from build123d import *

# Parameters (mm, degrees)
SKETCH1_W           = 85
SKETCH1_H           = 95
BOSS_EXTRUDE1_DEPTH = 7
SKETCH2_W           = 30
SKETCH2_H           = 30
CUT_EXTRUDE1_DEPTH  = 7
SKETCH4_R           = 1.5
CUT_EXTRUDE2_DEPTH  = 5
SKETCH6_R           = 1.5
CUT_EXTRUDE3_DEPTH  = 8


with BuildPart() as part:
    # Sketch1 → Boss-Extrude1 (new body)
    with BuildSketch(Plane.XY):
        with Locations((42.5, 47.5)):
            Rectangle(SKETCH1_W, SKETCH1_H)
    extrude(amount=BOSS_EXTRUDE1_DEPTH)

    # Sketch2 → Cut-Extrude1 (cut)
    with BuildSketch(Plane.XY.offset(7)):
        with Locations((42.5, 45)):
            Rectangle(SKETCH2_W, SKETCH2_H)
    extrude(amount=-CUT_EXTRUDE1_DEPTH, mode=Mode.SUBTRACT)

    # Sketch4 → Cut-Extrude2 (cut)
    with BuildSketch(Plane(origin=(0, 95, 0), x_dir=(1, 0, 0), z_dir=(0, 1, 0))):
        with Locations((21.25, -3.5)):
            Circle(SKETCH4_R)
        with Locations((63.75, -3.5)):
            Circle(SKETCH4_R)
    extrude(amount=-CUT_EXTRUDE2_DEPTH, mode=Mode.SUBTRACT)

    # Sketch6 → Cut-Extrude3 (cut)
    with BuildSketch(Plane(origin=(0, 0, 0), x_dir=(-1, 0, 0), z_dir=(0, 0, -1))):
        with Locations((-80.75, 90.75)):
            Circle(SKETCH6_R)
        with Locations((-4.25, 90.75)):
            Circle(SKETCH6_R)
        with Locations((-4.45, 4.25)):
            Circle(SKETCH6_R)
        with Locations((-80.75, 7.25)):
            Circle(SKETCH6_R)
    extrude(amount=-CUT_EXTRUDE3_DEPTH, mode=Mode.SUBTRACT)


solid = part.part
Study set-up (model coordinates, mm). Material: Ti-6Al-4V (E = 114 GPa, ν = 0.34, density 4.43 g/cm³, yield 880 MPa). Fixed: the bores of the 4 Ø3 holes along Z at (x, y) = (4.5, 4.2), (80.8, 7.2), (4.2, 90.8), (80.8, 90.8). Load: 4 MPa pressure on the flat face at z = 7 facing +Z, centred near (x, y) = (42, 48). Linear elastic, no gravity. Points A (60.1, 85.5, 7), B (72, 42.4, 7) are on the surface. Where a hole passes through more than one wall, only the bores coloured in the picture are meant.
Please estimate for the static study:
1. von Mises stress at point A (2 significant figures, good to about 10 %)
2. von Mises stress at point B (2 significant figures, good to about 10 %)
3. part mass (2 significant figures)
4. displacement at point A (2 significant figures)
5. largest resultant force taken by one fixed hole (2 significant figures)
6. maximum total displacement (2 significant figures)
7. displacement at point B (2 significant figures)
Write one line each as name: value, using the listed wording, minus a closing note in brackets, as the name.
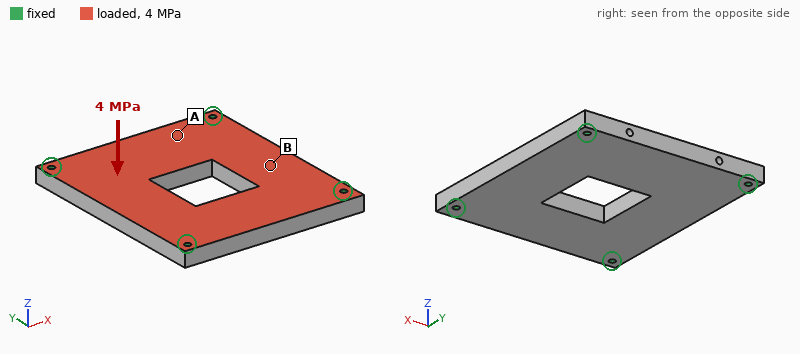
von Mises stress at point A: 110 MPa
von Mises stress at point B: 200 MPa
part mass: 220 g
displacement at point A: 0.20 mm
largest resultant force taken by one fixed hole: 7.5 kN
maximum total displacement: 0.54 mm
displacement at point B: 0.36 mm
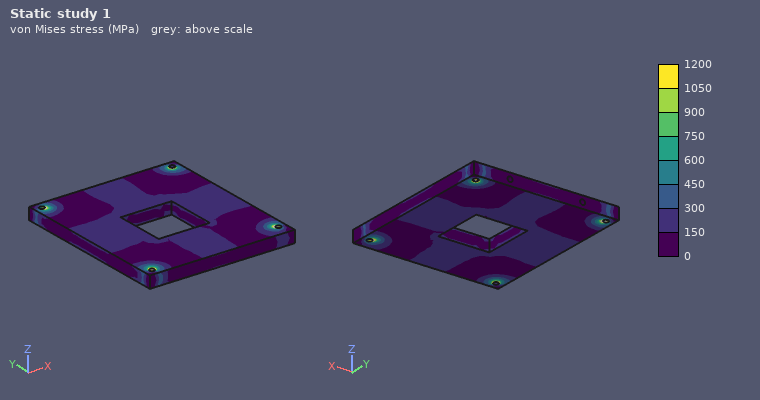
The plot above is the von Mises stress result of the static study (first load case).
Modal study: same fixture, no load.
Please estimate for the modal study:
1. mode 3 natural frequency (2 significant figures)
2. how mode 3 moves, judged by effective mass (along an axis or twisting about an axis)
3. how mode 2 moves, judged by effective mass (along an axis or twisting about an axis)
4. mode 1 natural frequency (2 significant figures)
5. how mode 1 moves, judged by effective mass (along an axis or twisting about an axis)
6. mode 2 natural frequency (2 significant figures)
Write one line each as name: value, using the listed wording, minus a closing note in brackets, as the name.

mode 3 natural frequency: 5500 Hz
how mode 3 moves, judged by effective mass: twisting about X
how mode 2 moves, judged by effective mass: twisting about Y
mode 1 natural frequency: 3100 Hz
how mode 1 moves, judged by effective mass: along Z
mode 2 natural frequency: 5000 Hz
